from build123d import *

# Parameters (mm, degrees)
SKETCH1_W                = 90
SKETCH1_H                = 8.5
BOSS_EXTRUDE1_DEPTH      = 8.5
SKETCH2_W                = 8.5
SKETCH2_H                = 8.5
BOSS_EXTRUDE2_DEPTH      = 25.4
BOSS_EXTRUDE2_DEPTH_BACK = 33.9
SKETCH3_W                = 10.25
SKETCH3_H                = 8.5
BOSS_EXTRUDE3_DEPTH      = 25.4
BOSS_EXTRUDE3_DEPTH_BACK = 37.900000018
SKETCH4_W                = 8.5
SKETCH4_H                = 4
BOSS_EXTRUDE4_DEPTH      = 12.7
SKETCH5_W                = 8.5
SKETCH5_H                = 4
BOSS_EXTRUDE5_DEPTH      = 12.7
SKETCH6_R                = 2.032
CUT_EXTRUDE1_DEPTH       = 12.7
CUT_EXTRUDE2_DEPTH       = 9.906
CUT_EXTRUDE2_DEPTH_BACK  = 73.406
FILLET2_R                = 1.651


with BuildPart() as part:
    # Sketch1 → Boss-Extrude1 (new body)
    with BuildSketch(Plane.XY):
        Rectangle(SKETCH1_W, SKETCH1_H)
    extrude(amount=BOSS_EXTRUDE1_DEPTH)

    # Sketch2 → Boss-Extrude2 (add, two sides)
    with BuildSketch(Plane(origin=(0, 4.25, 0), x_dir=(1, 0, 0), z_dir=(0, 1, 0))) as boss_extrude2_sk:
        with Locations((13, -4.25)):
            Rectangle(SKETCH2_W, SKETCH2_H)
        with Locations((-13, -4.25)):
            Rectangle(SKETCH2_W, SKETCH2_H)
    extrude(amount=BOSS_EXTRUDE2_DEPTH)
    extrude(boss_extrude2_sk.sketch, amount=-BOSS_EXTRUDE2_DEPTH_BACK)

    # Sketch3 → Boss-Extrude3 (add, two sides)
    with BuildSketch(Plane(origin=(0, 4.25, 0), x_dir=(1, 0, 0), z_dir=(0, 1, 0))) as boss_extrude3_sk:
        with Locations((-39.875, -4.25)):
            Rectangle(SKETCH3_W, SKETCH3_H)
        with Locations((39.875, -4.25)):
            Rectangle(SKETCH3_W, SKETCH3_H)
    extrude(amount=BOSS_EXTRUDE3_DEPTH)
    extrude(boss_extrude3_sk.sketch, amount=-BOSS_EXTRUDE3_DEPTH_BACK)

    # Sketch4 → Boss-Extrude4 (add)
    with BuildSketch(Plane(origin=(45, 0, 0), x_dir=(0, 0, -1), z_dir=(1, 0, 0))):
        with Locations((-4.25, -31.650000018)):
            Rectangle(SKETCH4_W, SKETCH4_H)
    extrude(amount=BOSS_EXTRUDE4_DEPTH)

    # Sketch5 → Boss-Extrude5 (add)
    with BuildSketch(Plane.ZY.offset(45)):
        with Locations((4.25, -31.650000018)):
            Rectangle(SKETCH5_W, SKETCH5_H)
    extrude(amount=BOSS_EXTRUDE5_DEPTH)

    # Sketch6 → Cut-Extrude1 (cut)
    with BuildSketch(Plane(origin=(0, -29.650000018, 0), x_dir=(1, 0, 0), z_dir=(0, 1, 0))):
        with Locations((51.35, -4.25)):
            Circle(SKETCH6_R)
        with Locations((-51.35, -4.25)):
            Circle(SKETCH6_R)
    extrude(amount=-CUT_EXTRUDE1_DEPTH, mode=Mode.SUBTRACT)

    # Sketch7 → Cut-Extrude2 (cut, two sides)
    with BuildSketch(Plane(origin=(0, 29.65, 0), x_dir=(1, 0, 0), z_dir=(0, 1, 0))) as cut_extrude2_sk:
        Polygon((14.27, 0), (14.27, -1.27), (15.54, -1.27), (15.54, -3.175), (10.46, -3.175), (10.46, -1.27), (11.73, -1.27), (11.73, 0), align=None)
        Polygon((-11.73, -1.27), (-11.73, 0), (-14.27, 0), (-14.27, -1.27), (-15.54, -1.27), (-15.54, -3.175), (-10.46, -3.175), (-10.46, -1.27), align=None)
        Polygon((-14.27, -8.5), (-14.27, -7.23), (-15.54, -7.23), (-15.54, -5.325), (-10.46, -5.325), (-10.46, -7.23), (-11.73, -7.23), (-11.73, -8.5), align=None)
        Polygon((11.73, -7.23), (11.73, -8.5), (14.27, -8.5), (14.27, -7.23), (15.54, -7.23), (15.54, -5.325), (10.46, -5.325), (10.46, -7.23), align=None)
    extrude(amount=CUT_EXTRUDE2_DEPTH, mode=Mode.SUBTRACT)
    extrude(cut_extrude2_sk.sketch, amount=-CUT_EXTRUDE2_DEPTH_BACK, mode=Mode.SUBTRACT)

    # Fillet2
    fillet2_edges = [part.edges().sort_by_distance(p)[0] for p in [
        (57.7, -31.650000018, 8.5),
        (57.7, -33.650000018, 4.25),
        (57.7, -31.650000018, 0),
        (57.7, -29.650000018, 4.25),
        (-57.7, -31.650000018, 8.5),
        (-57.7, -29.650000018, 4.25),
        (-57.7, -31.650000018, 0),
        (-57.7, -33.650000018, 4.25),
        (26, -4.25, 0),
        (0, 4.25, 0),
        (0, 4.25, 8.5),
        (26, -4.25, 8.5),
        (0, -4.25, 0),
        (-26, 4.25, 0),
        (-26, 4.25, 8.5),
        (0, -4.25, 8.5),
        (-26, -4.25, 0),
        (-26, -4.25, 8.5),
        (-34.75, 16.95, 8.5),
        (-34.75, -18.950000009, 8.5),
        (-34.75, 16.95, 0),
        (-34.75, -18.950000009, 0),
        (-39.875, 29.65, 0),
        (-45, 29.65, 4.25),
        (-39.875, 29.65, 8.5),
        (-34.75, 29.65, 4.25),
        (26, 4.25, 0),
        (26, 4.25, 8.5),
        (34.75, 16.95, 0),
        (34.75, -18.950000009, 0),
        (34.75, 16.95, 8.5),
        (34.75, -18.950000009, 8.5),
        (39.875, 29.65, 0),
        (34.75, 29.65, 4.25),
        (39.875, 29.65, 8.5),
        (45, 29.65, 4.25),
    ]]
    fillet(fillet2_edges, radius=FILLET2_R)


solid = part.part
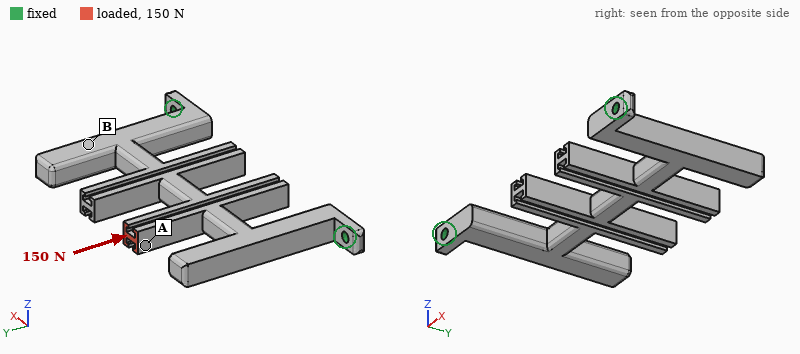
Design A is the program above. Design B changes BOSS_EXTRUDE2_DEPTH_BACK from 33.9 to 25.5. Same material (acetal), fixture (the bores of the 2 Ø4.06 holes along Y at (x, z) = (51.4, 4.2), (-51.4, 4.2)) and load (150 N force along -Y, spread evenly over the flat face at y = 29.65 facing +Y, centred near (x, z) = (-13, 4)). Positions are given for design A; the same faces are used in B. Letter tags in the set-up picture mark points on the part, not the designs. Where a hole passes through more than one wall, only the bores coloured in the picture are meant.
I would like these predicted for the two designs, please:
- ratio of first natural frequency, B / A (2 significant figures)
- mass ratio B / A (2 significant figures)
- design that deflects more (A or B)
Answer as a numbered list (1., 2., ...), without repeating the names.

1. 1.0
2. 0.96
3. A
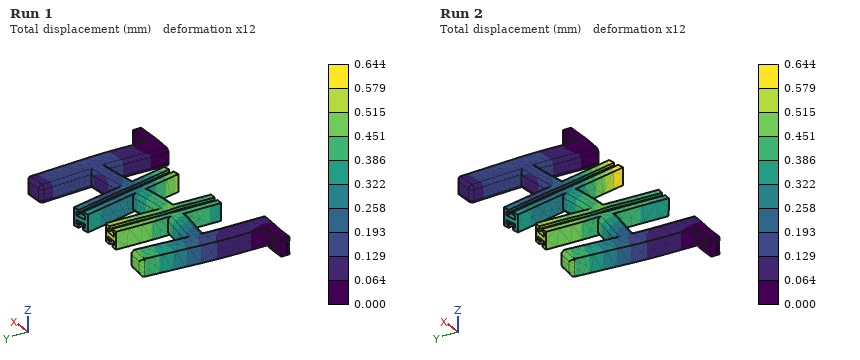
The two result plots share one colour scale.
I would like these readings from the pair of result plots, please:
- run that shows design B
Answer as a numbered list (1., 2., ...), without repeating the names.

1. Run 1
